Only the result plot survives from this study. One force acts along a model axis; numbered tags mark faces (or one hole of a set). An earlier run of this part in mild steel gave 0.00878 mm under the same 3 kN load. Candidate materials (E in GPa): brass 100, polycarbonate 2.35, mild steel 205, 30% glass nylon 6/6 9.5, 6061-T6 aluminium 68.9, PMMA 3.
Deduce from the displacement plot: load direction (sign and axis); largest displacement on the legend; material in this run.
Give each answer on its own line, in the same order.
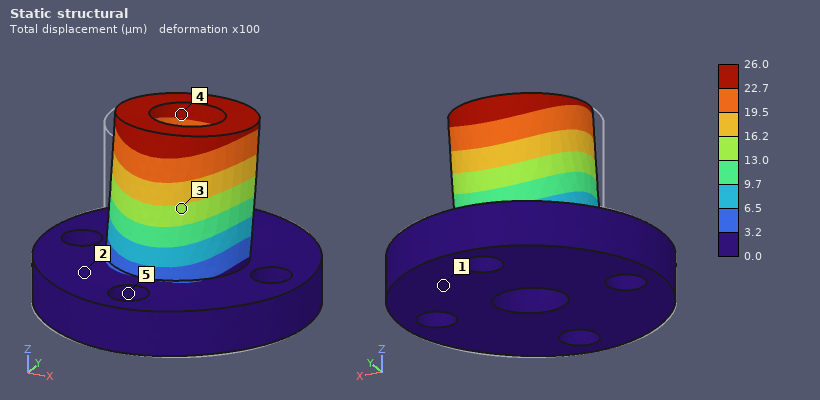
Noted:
+Y
26.0 µm
6061-T6 aluminium
